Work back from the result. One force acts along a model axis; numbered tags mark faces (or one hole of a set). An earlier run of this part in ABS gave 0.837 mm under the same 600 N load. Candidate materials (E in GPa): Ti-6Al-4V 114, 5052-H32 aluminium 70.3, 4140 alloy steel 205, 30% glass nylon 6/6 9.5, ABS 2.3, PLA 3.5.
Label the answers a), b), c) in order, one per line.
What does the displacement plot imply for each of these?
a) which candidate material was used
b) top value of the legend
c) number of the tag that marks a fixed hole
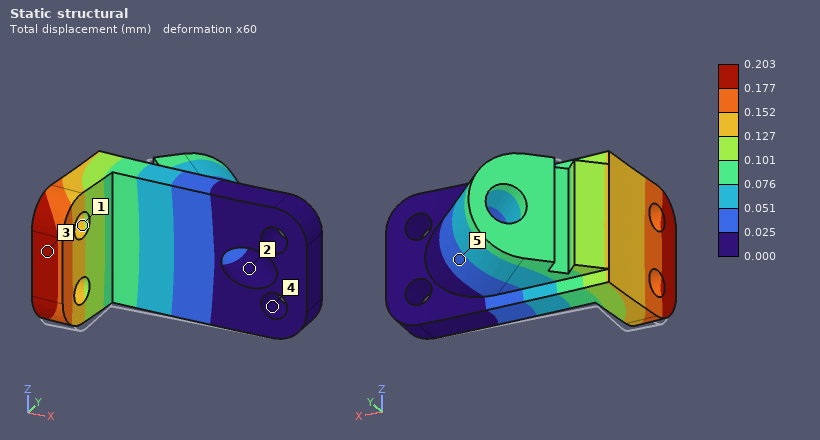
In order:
a) 30% glass nylon 6/6
b) 0.203 mm
c) 4
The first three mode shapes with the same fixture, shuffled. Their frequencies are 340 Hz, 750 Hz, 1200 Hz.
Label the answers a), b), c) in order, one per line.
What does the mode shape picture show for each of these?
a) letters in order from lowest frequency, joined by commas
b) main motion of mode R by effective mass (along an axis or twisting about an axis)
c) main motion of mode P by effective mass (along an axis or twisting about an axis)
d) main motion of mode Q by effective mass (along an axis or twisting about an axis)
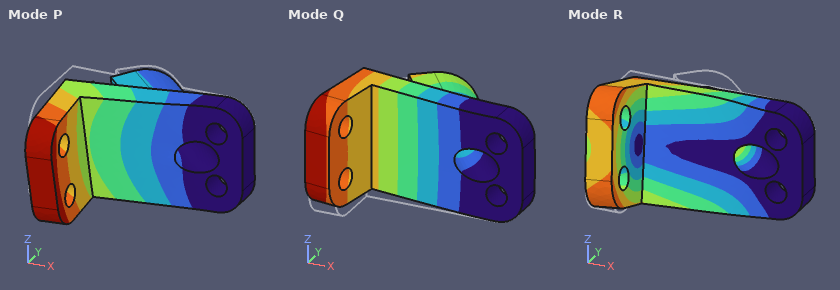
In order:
a) Q, P, R
b) along Z
c) along Z
d) along Y
